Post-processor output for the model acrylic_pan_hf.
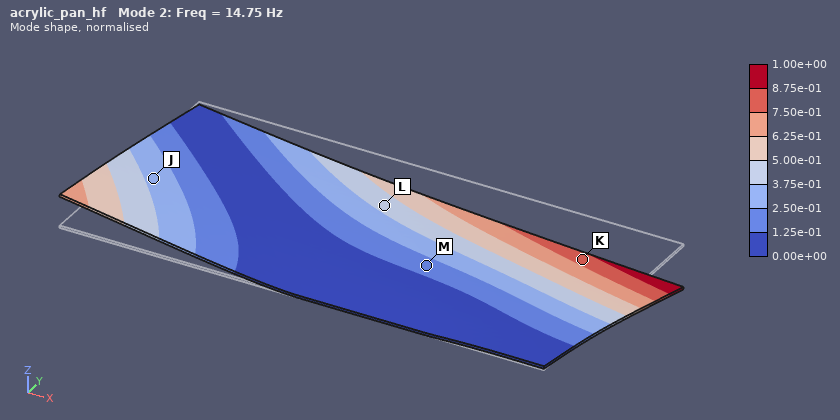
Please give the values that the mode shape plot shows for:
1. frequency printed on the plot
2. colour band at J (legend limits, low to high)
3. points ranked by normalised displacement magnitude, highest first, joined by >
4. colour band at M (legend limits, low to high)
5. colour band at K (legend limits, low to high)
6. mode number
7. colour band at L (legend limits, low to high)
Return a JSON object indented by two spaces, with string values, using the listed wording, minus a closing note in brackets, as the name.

{
  "frequency printed on the plot": "14.75 Hz",
  "colour band at J": "2.50e-01 to 3.75e-01",
  "points ranked by normalised displacement magnitude, highest first, joined by >": "K > L > J > M",
  "colour band at M": "1.25e-01 to 2.50e-01",
  "colour band at K": "7.50e-01 to 8.75e-01",
  "mode number": "2",
  "colour band at L": "3.75e-01 to 5.00e-01"
}
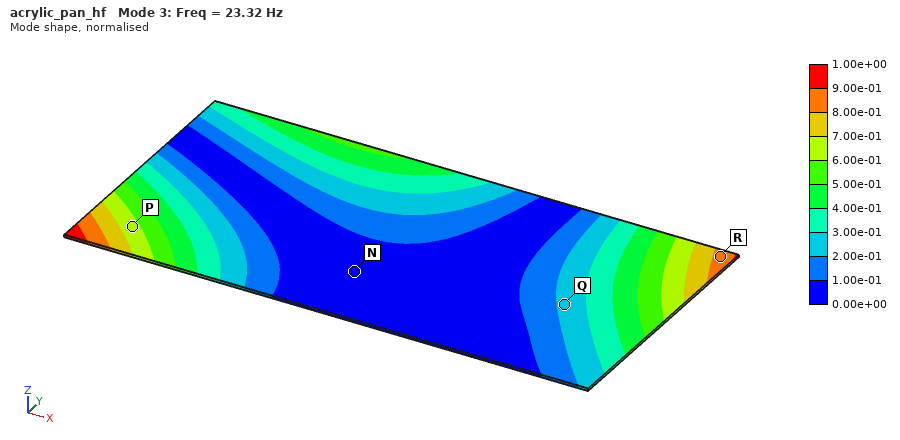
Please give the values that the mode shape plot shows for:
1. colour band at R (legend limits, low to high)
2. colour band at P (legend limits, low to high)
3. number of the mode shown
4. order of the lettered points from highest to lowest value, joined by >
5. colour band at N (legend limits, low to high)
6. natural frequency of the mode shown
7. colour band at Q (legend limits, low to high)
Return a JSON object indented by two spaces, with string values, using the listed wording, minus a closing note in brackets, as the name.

{
  "colour band at R": "8.00e-01 to 9.00e-01",
  "colour band at P": "6.00e-01 to 7.00e-01",
  "number of the mode shown": "3",
  "order of the lettered points from highest to lowest value, joined by >": "R > P > Q > N",
  "colour band at N": "0.00e+00 to 1.00e-01",
  "natural frequency of the mode shown": "23.32 Hz",
  "colour band at Q": "2.00e-01 to 3.00e-01"
}
